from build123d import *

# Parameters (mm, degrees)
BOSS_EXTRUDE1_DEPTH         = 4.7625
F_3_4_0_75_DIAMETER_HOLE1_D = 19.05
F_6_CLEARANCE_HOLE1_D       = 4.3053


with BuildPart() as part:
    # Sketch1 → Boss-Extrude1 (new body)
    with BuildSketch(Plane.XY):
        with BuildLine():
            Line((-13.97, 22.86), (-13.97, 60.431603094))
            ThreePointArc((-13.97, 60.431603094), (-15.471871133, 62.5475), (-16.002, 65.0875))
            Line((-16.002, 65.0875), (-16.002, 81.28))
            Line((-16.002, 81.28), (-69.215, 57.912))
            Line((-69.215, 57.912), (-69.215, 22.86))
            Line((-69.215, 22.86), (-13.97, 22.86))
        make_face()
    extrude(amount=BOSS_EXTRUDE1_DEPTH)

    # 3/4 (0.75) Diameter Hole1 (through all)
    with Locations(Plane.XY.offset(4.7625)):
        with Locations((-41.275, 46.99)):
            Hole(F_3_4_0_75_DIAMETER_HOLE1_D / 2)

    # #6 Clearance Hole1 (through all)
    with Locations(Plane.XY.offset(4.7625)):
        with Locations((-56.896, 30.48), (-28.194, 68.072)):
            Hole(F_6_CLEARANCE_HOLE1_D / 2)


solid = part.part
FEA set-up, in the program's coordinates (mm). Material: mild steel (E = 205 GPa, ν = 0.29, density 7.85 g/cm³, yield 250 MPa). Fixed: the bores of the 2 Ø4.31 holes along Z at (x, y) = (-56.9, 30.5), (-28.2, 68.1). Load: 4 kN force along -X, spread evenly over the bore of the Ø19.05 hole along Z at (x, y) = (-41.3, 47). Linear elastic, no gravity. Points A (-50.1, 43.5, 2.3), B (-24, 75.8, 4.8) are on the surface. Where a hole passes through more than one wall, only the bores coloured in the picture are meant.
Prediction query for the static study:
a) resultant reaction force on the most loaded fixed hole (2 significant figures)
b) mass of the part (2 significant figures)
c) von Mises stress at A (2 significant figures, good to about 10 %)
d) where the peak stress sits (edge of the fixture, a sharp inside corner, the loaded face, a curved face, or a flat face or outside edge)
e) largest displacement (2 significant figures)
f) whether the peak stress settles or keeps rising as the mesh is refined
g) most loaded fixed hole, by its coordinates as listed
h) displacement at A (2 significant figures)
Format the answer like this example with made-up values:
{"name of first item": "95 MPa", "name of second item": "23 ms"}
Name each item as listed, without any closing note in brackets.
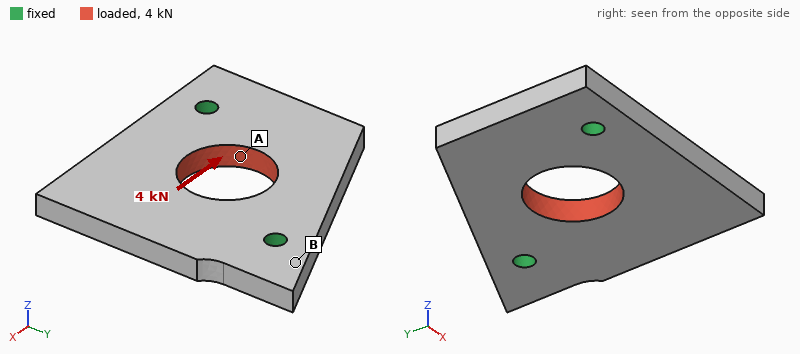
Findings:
{"resultant reaction force on the most loaded fixed hole": "2.2 kN", "mass of the part": "84 g", "von Mises stress at A": "22 MPa", "where the peak stress sits": "edge of the fixture", "largest displacement": "4.0 µm", "whether the peak stress settles or keeps rising as the mesh is refined": "keeps rising", "most loaded fixed hole, by its coordinates as listed": "(-56.9, 30.5)", "displacement at A": "2.9 µm"}
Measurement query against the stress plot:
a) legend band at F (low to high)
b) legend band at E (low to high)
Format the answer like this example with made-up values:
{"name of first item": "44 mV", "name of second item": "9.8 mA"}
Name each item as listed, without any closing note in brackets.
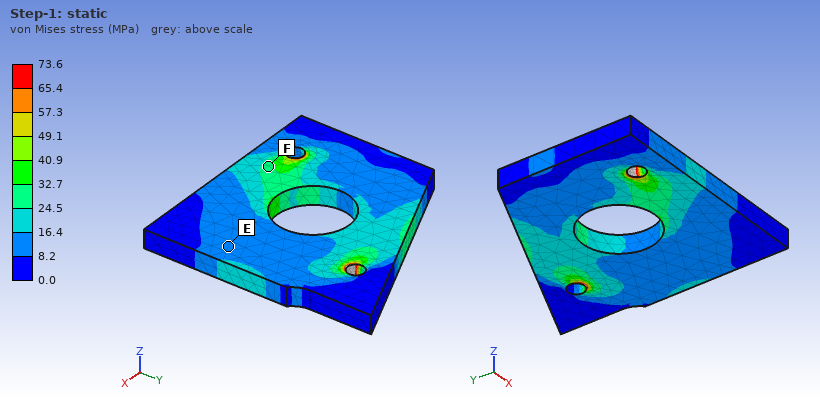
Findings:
{"legend band at F": "24.5 to 32.7 MPa", "legend band at E": "8.2 to 16.4 MPa"}
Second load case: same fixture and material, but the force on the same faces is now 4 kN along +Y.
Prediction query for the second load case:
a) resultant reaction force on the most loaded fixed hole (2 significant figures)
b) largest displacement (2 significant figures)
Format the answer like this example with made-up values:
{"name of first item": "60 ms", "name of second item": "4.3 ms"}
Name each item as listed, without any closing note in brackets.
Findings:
{"resultant reaction force on the most loaded fixed hole": "2.1 kN", "largest displacement": "3.7 µm"}
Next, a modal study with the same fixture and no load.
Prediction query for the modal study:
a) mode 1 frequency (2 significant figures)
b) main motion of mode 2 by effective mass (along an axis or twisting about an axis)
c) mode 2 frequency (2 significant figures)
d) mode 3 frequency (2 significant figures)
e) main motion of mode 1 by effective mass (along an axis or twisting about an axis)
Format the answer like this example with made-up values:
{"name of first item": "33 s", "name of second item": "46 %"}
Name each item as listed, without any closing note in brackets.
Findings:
{"mode 1 frequency": "3400 Hz", "main motion of mode 2 by effective mass": "along Z", "mode 2 frequency": "6200 Hz", "mode 3 frequency": "11 kHz", "main motion of mode 1 by effective mass": "along Z"}
